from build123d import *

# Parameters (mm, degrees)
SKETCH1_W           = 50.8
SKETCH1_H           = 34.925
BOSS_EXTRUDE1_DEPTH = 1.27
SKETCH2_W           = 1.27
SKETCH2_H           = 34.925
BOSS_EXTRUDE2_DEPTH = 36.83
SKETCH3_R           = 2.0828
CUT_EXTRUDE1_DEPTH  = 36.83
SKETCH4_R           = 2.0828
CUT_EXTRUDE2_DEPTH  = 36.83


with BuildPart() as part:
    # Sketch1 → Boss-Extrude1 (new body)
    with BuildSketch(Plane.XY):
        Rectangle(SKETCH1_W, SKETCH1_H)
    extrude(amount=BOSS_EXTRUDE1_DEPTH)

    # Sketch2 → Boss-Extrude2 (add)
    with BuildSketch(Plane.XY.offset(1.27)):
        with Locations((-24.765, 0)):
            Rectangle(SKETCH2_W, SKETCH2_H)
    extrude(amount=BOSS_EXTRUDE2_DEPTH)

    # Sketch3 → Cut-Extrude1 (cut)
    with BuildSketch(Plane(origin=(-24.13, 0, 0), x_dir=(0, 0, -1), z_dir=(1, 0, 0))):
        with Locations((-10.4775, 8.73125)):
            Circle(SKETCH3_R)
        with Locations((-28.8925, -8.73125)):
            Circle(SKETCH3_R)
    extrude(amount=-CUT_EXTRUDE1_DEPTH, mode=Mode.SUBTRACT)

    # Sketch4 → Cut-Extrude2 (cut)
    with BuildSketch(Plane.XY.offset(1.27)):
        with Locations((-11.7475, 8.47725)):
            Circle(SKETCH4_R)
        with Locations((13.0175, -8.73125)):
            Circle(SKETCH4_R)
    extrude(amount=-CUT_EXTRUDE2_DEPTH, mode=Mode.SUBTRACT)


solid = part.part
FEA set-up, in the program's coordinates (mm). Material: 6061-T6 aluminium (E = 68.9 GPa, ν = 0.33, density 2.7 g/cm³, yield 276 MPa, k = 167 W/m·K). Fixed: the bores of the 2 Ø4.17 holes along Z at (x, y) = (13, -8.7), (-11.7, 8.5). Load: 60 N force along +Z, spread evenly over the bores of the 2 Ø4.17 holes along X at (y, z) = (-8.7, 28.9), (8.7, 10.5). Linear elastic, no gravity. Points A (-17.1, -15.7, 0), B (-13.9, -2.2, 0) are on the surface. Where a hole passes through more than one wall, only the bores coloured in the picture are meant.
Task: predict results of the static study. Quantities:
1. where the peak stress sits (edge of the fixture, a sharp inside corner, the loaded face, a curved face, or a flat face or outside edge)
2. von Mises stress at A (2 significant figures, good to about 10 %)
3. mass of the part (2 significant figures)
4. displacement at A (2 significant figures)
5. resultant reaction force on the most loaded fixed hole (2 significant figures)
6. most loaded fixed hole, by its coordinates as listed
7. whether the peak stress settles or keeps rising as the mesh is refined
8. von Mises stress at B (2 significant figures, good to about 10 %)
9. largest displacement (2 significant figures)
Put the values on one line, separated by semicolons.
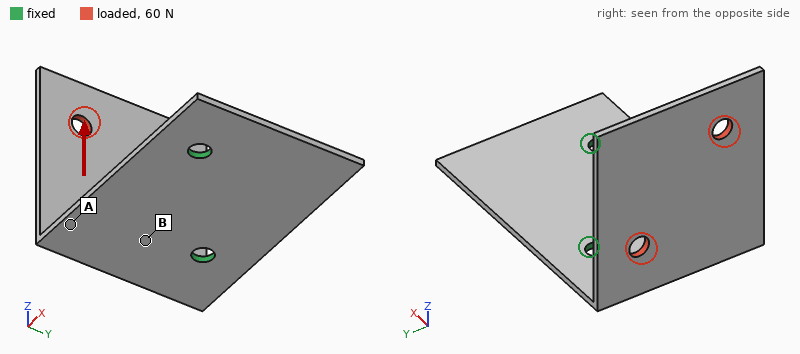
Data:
edge of the fixture; 23 MPa; 10 g; 0.21 mm; 64 N; (-11.7, 8.5); keeps rising; 48 MPa; 0.74 mm
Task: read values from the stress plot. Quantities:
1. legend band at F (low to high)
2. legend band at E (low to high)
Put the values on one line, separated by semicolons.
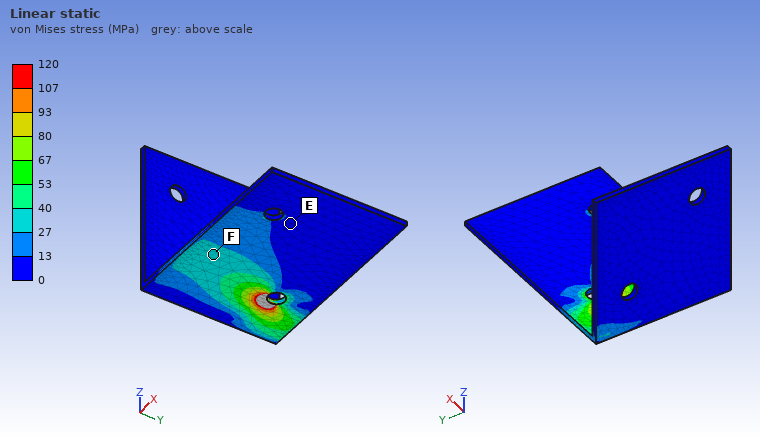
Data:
27 to 40 MPa; 0 to 13 MPa
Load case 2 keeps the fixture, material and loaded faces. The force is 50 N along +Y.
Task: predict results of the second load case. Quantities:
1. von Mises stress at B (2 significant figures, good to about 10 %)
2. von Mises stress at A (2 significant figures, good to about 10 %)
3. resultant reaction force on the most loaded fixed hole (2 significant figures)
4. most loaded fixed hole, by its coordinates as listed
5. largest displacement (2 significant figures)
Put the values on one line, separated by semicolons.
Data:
38 MPa; 29 MPa; 61 N; (-11.7, 8.5); 0.82 mm
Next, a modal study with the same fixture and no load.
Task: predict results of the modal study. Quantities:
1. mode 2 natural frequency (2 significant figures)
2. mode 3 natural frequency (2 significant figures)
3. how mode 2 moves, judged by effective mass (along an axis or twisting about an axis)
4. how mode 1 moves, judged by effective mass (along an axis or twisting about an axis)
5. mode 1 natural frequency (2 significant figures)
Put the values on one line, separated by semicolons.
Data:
730 Hz; 1700 Hz; along Y; along X; 460 Hz
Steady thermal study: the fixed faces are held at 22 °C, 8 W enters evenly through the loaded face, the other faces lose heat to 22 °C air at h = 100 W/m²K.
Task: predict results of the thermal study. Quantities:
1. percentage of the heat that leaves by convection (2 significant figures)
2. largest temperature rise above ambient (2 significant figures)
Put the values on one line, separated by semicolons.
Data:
60 %; 23 K
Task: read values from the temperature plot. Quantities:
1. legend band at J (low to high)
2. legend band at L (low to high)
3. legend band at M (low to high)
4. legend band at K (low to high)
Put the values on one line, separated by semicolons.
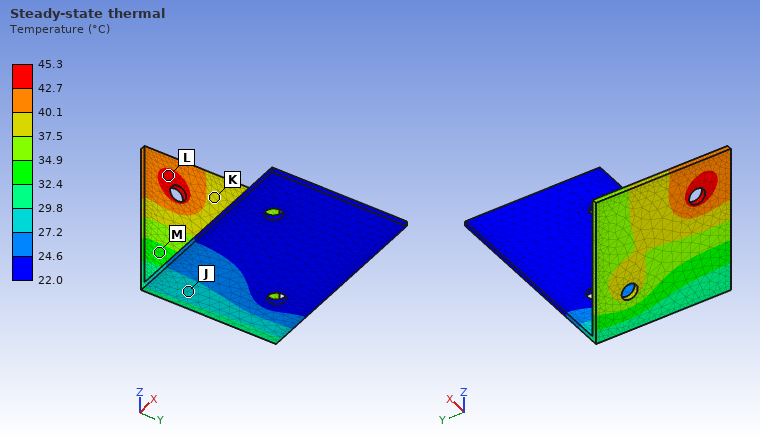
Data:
27.2 to 29.8 °C; 42.7 to 45.3 °C; 32.4 to 34.9 °C; 37.5 to 40.1 °C
